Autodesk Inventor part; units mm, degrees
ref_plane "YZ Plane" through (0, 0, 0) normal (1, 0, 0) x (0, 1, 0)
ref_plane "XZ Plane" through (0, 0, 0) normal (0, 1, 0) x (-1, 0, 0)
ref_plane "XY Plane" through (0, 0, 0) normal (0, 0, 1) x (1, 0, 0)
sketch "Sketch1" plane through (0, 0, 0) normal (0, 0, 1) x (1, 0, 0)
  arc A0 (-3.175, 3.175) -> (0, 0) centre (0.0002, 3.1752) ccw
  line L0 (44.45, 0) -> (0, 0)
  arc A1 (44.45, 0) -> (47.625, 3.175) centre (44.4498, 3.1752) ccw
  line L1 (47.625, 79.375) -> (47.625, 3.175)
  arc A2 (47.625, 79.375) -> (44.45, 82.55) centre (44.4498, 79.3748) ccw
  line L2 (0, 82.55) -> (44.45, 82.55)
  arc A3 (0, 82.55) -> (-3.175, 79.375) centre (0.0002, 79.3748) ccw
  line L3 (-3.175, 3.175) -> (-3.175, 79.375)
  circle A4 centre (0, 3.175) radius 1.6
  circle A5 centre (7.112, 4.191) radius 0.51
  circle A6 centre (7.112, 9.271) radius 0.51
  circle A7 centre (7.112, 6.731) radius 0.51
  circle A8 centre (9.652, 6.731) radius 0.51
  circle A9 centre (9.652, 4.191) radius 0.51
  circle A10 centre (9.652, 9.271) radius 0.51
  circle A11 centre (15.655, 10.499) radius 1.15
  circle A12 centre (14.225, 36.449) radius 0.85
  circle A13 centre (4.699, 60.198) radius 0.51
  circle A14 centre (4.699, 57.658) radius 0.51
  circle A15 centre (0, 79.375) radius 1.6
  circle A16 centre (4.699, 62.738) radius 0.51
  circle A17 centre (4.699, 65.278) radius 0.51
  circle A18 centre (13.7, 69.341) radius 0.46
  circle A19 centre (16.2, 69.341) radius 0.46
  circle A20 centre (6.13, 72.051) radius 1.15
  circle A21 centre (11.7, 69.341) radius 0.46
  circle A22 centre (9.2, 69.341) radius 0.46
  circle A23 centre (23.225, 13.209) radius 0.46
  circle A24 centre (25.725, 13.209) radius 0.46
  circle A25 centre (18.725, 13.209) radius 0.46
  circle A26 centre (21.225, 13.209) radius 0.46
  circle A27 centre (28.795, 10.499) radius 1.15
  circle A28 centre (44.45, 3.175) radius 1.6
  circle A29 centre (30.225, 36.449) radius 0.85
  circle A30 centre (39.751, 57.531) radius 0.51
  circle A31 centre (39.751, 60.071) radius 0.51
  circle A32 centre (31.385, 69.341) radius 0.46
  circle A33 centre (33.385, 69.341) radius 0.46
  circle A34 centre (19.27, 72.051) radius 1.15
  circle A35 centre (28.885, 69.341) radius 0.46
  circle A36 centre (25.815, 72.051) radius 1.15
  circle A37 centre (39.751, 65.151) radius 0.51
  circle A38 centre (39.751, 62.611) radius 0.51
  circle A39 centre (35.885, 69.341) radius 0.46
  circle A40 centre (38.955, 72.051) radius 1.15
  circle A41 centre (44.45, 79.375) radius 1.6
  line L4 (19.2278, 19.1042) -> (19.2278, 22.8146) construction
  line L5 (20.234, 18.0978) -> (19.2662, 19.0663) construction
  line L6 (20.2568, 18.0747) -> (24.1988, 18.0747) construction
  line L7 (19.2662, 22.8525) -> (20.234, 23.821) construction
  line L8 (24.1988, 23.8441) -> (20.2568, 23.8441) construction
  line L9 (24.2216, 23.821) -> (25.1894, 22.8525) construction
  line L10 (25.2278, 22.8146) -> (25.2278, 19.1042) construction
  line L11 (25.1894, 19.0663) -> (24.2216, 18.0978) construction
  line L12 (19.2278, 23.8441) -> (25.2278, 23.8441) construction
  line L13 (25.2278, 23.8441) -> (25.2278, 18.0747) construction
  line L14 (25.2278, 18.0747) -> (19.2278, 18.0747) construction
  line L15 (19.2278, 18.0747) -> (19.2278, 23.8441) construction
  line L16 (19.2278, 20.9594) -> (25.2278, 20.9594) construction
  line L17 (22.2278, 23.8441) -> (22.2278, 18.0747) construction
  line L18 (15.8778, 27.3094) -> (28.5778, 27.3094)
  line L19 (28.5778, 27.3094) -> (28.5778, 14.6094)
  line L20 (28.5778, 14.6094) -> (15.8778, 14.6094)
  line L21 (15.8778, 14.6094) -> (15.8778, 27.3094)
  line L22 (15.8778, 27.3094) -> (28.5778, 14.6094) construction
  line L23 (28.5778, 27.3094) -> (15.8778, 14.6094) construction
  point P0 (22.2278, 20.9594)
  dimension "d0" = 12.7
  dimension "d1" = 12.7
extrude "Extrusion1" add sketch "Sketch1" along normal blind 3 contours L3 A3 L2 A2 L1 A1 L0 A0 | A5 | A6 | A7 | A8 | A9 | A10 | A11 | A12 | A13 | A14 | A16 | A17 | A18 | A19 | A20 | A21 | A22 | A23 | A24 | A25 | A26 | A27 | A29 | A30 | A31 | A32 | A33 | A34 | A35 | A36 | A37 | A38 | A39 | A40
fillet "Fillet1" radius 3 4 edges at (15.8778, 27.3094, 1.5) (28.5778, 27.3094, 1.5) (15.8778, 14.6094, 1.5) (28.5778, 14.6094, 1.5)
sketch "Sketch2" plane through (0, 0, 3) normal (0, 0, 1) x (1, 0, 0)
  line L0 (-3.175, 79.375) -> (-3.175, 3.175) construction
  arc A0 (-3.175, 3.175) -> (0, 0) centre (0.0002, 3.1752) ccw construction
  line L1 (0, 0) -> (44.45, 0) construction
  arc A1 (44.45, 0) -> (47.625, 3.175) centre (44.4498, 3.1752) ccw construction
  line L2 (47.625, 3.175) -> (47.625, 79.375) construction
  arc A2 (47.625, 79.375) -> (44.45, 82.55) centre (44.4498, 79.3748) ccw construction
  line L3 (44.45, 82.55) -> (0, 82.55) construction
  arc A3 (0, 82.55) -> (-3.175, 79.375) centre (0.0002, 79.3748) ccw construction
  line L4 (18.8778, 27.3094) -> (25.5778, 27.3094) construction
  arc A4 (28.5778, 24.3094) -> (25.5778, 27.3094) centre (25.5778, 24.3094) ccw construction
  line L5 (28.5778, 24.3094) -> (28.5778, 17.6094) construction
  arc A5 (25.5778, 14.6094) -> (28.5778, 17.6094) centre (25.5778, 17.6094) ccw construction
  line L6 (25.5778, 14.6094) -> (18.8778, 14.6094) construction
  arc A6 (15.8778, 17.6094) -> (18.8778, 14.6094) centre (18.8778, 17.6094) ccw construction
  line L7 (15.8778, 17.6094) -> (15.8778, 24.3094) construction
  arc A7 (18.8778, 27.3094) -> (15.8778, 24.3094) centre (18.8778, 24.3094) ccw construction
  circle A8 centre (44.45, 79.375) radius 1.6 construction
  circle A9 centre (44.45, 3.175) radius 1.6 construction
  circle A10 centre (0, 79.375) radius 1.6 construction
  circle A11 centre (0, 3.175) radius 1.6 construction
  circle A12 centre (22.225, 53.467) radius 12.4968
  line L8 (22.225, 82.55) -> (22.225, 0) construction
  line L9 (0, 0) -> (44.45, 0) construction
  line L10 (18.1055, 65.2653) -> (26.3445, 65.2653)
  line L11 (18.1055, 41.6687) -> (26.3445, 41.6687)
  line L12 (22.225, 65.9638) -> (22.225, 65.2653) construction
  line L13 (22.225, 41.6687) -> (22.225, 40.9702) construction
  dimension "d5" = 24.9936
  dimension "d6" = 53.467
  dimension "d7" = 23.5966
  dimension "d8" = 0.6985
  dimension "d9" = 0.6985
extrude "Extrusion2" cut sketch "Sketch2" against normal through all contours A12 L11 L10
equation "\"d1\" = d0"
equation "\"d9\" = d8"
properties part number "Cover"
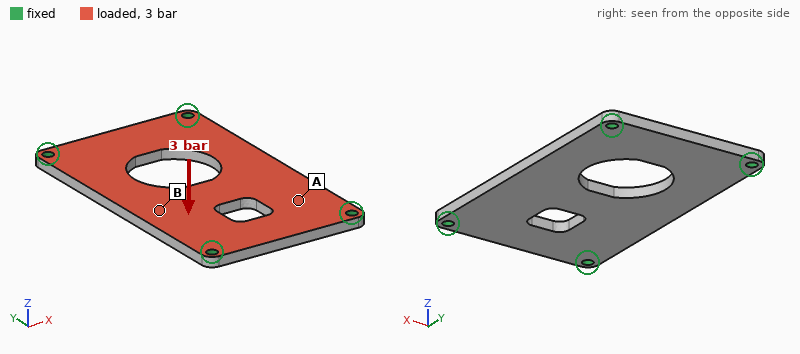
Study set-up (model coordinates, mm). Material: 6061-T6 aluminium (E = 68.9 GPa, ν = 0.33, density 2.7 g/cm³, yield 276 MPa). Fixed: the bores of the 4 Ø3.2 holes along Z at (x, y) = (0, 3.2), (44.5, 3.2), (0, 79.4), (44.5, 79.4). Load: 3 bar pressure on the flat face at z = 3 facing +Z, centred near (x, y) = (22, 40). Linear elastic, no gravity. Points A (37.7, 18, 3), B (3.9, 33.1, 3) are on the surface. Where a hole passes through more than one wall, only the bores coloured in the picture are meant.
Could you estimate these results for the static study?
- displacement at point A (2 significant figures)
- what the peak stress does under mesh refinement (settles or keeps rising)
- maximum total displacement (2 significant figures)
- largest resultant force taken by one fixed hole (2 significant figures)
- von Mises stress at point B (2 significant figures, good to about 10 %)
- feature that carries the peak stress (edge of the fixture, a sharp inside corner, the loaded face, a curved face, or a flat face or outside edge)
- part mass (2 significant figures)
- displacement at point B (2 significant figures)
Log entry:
0.11 mm
keeps rising
0.27 mm
270 N
44 MPa
edge of the fixture
28 g
0.21 mm
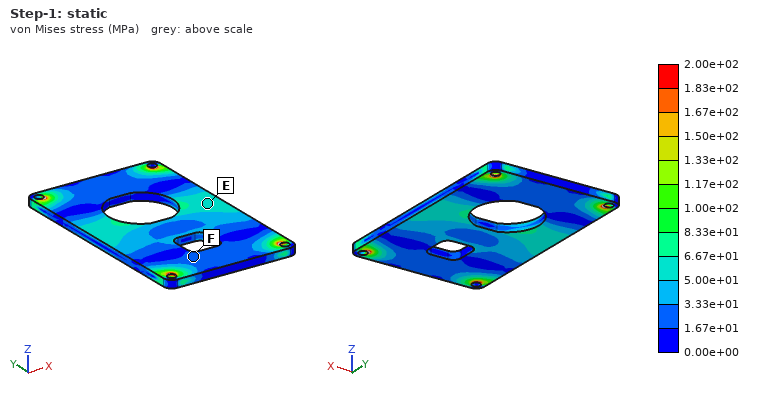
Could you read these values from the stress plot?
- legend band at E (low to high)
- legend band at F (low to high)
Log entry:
5.00e+01 to 6.67e+01 MPa
1.67e+01 to 3.33e+01 MPa
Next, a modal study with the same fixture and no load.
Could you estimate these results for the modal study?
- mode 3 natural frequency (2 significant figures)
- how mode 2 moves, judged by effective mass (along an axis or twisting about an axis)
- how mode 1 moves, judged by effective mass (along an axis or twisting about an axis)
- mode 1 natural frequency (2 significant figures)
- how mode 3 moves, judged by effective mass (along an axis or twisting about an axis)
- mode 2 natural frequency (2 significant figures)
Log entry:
5800 Hz
twisting about Y
along Z
2300 Hz
twisting about X
3500 Hz
